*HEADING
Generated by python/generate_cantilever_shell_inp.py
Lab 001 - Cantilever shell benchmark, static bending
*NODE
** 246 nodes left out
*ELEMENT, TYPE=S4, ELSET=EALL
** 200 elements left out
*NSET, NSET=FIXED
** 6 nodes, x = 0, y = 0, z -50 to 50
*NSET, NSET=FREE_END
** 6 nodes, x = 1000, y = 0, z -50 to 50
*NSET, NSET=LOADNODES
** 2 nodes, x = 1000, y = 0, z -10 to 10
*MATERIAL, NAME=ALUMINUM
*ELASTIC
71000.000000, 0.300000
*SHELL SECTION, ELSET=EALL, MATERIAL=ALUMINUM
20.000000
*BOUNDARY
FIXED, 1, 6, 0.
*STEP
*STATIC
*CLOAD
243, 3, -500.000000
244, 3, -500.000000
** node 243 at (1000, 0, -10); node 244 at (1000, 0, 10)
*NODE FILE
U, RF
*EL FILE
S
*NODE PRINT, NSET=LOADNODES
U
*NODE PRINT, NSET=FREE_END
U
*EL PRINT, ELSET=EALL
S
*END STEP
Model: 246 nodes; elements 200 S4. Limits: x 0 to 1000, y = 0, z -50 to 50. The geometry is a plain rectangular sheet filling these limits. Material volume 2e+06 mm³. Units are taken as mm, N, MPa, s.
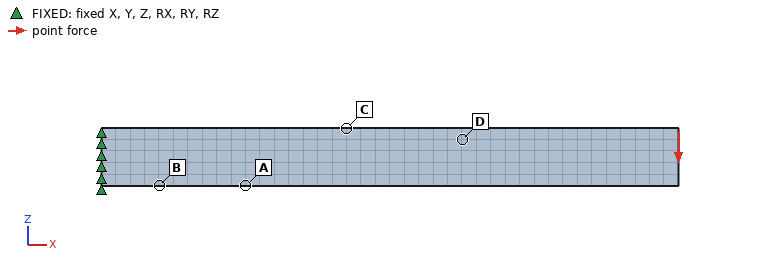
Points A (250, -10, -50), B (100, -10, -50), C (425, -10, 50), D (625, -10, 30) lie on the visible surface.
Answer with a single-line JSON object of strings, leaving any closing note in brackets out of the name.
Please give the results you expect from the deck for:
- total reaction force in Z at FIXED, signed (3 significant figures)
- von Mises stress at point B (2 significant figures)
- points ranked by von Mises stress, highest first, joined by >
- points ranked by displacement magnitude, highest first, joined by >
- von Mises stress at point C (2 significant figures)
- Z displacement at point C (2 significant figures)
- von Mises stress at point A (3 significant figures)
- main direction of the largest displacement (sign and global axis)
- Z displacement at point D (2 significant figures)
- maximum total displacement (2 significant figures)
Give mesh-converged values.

{"total reaction force in Z at FIXED, signed": "1000 N", "von Mises stress at point B": "27 MPa", "points ranked by von Mises stress, highest first, joined by >": "B > A > C > D", "points ranked by displacement magnitude, highest first, joined by >": "D > C > A > B", "von Mises stress at point C": "17 MPa", "Z displacement at point C": "-0.66 mm", "von Mises stress at point A": "22.5 MPa", "main direction of the largest displacement": "-Z", "Z displacement at point D": "-1.3 mm", "maximum total displacement": "2.8 mm"}
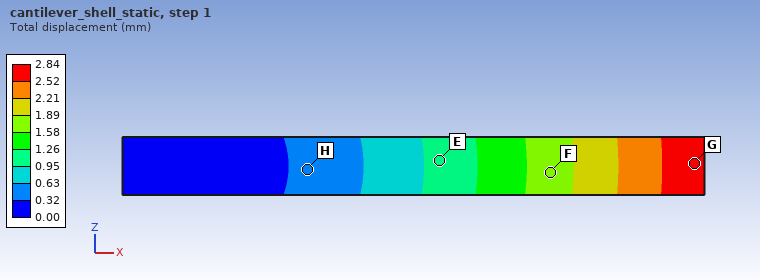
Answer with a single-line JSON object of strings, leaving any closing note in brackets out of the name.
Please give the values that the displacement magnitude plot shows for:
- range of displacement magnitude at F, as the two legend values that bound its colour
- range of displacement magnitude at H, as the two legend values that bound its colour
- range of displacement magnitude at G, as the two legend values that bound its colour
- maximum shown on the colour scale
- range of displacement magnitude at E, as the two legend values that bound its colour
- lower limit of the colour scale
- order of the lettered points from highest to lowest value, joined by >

{"range of displacement magnitude at F, as the two legend values that bound its colour": "1.58 to 1.89 mm", "range of displacement magnitude at H, as the two legend values that bound its colour": "0.32 to 0.63 mm", "range of displacement magnitude at G, as the two legend values that bound its colour": "2.52 to 2.84 mm", "maximum shown on the colour scale": "2.84 mm", "range of displacement magnitude at E, as the two legend values that bound its colour": "0.95 to 1.26 mm", "lower limit of the colour scale": "0.00 mm", "order of the lettered points from highest to lowest value, joined by >": "G > F > E > H"}
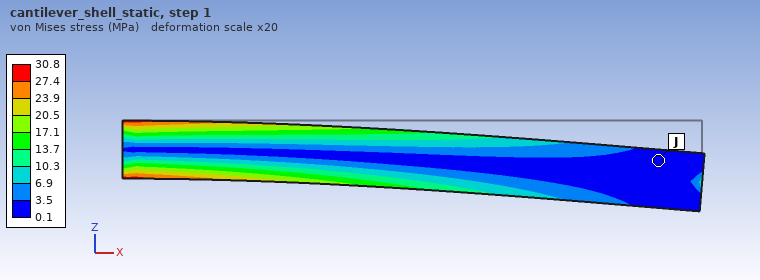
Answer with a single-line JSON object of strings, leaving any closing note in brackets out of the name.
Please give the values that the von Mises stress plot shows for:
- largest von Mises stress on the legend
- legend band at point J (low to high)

{"largest von Mises stress on the legend": "30.8 MPa", "legend band at point J": "0.1 to 3.5 MPa"}
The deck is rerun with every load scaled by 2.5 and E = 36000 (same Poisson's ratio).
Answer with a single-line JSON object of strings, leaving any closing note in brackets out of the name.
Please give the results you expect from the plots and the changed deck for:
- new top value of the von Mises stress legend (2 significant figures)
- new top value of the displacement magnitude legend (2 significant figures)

{"new top value of the von Mises stress legend": "77 MPa", "new top value of the displacement magnitude legend": "14 mm"}
